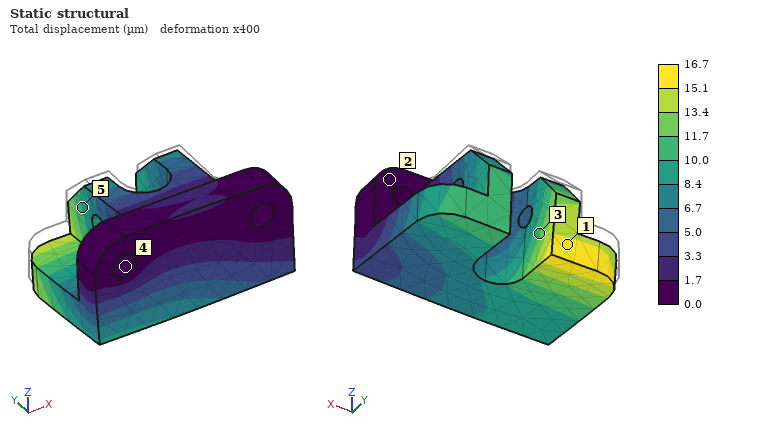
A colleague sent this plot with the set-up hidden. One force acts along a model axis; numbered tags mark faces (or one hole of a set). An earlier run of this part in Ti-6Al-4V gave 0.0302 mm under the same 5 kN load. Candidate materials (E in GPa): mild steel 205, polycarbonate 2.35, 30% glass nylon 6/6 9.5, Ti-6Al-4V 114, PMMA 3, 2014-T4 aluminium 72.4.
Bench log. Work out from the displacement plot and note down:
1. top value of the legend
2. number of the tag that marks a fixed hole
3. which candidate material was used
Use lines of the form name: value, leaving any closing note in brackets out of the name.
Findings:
top value of the legend: 16.7 µm
number of the tag that marks a fixed hole: 4
which candidate material was used: mild steel
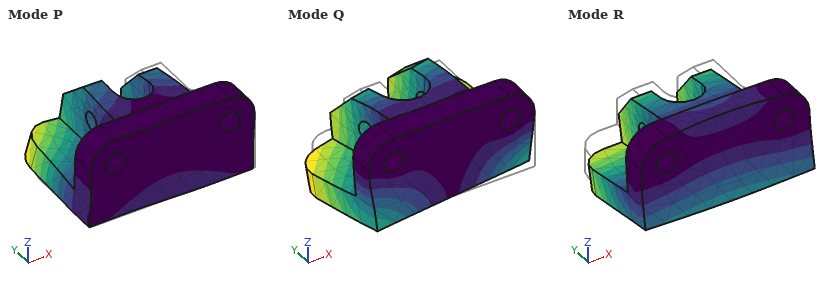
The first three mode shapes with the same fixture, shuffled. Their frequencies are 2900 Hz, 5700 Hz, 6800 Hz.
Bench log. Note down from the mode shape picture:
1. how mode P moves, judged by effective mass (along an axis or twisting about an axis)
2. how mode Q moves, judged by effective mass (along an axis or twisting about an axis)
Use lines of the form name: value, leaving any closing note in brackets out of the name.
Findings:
how mode P moves, judged by effective mass: along X
how mode Q moves, judged by effective mass: along X
